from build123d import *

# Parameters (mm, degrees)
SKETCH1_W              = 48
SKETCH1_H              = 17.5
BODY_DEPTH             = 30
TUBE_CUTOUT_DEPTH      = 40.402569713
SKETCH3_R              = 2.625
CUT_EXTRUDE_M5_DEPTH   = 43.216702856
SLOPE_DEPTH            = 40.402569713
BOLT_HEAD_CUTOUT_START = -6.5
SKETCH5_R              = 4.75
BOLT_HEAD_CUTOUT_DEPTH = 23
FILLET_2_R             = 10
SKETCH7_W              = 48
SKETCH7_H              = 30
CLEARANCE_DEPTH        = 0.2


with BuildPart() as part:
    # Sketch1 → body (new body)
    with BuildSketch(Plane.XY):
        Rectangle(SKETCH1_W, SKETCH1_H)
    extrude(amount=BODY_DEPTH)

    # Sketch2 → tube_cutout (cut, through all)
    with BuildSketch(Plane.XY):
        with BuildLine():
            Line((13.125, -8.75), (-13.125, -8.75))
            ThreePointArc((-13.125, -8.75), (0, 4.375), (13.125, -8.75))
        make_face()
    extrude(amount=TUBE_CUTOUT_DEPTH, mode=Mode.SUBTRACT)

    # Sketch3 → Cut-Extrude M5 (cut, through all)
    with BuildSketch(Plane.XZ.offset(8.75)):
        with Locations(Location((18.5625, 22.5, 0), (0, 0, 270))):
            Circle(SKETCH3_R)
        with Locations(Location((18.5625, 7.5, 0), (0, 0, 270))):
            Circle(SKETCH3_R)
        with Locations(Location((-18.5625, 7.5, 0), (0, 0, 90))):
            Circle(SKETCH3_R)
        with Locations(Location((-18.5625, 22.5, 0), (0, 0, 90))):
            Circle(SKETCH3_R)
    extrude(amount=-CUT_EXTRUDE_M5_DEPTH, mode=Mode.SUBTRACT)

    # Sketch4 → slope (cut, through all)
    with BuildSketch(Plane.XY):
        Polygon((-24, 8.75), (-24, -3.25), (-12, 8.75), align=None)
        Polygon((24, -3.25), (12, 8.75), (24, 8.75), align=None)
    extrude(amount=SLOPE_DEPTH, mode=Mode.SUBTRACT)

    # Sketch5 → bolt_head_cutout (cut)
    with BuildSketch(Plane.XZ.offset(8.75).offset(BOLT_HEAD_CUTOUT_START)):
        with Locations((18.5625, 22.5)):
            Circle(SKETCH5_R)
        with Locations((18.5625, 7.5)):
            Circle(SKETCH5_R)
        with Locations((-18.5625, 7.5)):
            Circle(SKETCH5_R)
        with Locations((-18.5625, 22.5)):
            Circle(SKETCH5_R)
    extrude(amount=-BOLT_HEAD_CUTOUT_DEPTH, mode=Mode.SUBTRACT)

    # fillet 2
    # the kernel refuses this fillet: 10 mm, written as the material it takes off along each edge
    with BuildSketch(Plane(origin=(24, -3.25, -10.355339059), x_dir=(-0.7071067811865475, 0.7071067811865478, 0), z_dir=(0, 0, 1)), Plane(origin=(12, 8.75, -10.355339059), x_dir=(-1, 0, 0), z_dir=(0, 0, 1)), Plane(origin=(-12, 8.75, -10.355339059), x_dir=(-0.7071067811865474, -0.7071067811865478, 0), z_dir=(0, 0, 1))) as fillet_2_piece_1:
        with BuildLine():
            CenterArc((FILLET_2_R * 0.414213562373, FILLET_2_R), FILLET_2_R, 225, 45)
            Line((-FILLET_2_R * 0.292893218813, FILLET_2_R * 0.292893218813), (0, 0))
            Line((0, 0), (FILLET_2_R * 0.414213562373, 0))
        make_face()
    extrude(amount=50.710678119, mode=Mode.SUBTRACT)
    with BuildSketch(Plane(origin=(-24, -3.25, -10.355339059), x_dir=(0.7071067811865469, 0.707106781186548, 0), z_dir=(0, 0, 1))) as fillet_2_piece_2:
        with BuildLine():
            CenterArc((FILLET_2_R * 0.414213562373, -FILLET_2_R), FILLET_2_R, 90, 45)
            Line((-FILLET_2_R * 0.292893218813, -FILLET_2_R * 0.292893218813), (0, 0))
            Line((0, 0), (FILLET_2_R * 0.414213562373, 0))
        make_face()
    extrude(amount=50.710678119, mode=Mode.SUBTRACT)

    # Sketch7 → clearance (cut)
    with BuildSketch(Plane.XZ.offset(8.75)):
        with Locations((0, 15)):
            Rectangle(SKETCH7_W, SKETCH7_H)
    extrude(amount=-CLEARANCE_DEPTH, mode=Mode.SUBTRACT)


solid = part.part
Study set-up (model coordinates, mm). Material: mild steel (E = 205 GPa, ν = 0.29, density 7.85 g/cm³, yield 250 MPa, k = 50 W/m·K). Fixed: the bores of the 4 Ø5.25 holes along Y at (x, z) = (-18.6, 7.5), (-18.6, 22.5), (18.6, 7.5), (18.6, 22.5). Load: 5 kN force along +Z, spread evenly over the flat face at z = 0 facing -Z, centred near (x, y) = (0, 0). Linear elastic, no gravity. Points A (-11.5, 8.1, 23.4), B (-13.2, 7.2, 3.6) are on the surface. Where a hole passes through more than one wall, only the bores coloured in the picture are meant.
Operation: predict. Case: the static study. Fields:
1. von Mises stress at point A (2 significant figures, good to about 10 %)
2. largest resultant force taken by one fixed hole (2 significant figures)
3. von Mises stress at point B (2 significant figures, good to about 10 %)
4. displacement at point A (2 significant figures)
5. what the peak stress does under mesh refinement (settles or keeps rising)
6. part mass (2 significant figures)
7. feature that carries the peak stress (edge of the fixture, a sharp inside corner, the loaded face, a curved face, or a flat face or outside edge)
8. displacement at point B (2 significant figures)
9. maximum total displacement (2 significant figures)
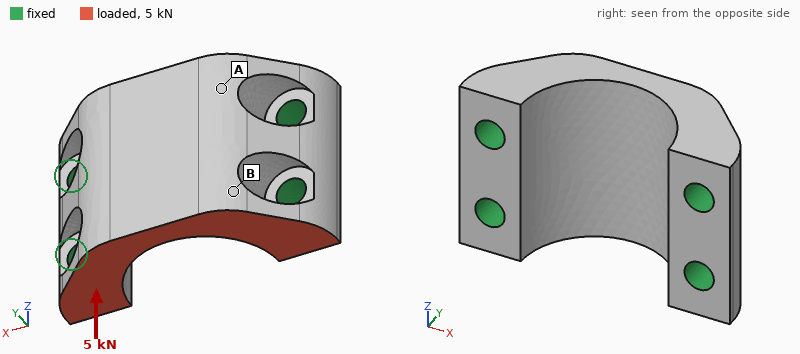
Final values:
9.5 MPa
2.0 kN
19 MPa
2.4 µm
keeps rising
83 g
edge of the fixture
3.5 µm
4.3 µm
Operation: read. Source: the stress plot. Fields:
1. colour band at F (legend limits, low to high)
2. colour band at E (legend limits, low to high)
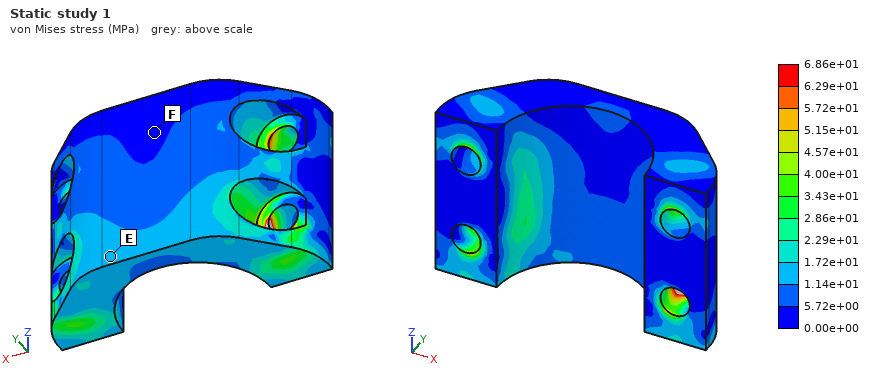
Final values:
0.00e+00 to 5.72e+00 MPa
1.14e+01 to 1.72e+01 MPa
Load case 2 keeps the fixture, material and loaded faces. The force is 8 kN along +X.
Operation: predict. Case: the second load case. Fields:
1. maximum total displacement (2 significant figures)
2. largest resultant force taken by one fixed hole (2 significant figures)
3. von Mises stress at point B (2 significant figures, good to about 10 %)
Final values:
13 µm
3.5 kN
57 MPa
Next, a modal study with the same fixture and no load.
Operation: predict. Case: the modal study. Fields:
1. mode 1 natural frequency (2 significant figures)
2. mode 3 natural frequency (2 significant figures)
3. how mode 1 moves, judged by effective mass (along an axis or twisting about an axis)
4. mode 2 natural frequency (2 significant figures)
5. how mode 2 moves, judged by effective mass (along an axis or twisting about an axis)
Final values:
23 kHz
30 kHz
along Z
26 kHz
along X
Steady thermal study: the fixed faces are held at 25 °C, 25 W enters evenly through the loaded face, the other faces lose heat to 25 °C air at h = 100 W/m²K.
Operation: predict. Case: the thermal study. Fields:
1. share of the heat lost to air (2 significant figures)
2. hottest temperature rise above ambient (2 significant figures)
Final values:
10 %
21 K
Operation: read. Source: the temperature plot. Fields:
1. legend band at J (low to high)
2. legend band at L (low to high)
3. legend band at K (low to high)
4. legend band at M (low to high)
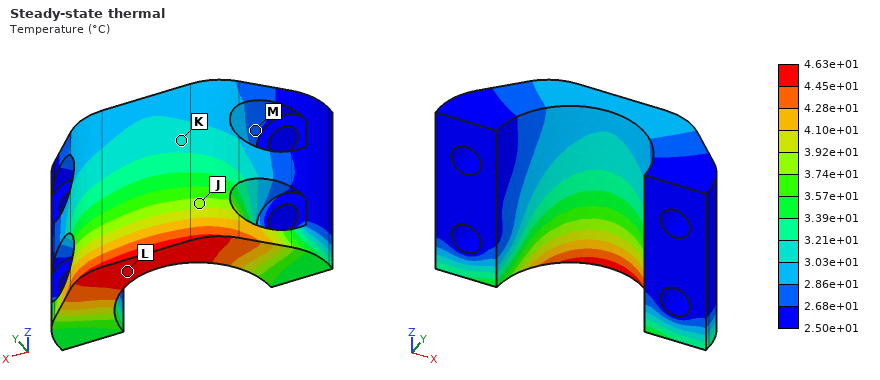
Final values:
3.74e+01 to 3.92e+01 °C
4.45e+01 to 4.63e+01 °C
3.03e+01 to 3.21e+01 °C
2.68e+01 to 2.86e+01 °C
